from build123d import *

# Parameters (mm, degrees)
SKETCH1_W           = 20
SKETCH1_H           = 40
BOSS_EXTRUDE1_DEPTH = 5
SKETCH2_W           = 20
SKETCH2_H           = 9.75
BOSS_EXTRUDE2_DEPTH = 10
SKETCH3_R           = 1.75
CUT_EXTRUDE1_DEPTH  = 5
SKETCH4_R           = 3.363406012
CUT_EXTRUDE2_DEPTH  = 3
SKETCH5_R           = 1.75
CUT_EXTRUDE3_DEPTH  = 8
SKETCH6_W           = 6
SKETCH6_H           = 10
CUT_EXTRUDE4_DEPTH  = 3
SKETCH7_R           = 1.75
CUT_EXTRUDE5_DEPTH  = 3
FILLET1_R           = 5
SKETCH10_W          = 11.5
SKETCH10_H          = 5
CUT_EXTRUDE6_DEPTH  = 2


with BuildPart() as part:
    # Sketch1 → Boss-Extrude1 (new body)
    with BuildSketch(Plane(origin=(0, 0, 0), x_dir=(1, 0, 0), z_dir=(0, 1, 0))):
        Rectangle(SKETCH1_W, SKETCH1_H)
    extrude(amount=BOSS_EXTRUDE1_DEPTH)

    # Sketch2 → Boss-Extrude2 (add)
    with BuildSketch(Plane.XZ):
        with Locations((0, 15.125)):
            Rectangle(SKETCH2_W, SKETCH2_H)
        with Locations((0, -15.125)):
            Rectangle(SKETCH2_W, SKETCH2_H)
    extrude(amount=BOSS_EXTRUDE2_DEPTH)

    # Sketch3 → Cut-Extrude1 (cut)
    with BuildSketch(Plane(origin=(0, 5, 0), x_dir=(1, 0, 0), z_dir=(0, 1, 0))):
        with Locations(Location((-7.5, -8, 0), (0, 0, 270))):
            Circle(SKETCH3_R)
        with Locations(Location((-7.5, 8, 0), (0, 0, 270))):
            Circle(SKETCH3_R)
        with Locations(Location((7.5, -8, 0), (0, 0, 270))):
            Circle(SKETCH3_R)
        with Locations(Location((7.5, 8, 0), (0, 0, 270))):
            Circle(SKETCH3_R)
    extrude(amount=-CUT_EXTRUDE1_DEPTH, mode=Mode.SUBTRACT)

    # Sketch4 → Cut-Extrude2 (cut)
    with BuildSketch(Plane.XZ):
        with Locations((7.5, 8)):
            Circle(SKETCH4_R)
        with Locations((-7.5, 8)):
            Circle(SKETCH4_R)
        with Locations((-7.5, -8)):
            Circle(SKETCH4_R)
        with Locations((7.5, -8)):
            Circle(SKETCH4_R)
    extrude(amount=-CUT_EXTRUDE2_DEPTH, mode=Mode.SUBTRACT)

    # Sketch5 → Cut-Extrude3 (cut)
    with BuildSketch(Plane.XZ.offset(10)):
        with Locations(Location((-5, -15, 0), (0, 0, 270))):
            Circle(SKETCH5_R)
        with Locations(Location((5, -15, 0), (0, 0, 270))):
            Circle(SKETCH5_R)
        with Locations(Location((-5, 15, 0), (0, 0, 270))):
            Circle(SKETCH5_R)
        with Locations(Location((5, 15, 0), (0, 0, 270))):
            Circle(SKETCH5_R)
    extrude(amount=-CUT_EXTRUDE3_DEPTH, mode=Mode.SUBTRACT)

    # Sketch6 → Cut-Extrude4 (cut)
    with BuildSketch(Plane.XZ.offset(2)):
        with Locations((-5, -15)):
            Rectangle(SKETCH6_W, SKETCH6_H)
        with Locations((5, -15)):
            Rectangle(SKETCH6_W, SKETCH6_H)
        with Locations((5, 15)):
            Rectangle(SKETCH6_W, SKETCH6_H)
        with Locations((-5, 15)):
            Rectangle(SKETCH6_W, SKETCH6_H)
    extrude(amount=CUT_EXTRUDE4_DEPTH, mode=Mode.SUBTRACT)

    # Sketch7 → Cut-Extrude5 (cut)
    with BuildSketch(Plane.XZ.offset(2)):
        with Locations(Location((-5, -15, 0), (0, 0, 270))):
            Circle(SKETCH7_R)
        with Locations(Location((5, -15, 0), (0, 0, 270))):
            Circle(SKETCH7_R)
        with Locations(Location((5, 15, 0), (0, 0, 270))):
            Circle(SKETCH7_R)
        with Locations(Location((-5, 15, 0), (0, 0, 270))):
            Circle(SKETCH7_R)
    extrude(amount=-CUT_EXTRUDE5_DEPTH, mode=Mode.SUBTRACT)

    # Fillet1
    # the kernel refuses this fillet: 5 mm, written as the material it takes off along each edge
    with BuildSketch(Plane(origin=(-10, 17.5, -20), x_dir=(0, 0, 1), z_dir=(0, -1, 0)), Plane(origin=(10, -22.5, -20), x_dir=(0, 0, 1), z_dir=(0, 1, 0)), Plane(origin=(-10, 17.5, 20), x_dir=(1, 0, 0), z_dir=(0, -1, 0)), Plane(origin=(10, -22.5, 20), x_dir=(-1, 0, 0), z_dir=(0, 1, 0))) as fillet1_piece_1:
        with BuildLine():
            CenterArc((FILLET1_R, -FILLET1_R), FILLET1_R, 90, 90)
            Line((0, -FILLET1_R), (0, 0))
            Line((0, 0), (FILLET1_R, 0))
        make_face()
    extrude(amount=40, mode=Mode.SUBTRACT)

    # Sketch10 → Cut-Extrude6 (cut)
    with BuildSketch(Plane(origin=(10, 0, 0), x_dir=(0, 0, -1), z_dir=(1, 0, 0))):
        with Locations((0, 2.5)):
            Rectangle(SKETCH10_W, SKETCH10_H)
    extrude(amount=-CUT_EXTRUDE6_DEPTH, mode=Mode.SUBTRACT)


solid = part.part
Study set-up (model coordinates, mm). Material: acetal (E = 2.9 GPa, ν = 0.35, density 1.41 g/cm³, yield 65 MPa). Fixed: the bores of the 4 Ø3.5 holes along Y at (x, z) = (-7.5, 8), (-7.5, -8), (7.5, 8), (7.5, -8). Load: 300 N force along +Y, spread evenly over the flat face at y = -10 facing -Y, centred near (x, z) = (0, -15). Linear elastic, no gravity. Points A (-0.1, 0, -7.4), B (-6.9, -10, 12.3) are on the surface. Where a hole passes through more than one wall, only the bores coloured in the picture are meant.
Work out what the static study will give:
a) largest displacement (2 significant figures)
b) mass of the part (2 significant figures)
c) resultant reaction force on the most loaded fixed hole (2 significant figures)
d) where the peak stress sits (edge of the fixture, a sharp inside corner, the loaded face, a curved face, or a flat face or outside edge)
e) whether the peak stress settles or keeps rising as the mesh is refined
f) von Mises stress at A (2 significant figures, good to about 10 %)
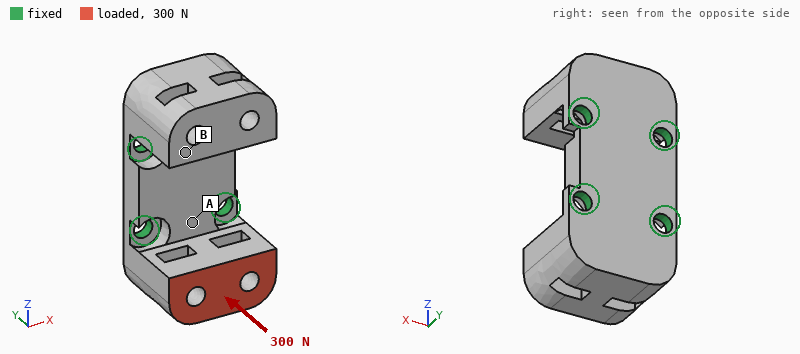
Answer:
0.46 mm
8.5 g
210 N
edge of the fixture
keeps rising
20 MPa
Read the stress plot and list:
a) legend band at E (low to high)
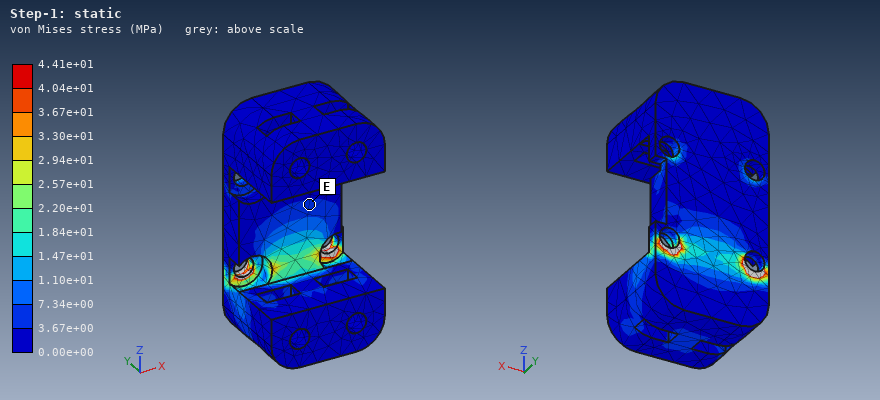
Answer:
3.67e+00 to 7.34e+00 MPa
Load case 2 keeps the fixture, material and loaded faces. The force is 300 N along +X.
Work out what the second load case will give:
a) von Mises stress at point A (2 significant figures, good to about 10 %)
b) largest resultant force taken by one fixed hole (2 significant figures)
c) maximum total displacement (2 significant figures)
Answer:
15 MPa
340 N
0.32 mm
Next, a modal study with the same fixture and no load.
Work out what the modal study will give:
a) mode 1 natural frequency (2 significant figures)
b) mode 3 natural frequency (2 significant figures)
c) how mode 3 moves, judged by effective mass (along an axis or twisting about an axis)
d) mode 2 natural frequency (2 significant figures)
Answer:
2300 Hz
4700 Hz
along X
2300 Hz
